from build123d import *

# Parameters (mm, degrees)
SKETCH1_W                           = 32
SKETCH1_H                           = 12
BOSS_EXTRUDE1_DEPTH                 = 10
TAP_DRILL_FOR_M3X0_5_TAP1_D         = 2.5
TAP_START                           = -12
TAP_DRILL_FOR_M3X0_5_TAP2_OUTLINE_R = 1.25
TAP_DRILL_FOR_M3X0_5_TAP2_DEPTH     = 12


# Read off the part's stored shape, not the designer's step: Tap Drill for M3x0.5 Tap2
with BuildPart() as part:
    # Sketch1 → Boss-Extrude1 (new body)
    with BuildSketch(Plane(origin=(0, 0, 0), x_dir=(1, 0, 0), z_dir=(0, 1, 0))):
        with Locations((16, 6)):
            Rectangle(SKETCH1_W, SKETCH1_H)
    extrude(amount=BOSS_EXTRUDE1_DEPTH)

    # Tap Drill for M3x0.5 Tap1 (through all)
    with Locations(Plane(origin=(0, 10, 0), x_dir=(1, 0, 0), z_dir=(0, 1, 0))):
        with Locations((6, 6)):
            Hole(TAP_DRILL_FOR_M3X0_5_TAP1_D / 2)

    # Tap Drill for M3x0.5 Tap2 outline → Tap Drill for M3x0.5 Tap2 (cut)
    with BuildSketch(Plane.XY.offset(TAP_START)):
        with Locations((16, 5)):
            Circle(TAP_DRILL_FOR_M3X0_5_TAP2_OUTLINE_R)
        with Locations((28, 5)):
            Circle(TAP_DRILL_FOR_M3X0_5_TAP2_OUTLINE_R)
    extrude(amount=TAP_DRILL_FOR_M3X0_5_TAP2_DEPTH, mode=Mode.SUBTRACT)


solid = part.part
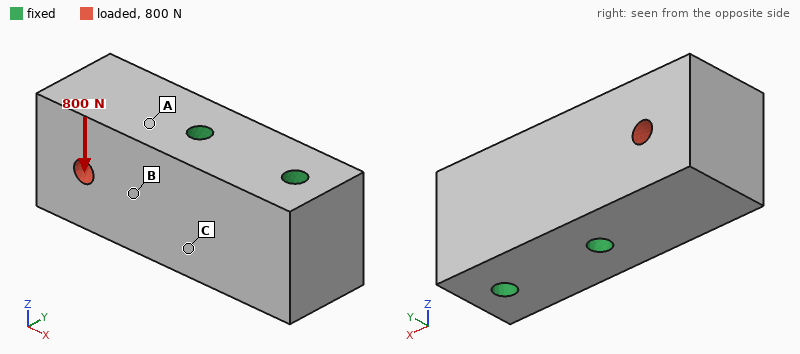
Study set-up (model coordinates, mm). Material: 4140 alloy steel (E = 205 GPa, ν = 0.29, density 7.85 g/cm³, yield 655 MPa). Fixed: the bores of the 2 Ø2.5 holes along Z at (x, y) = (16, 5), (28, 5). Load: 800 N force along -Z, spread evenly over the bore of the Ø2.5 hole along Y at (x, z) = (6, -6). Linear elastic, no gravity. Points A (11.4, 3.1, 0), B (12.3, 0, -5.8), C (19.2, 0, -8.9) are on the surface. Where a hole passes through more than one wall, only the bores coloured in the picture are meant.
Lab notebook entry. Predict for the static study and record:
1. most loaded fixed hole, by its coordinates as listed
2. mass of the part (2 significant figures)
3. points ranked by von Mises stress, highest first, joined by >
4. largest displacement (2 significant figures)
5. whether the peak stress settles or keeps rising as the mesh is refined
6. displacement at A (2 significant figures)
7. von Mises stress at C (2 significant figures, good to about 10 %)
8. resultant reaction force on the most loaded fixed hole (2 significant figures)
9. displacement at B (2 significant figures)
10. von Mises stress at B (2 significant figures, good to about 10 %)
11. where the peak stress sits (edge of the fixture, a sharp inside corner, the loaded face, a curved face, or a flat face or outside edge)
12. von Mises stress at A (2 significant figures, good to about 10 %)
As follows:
(16, 5)
29 g
A > B > C
3.2 µm
keeps rising
1.1 µm
5.1 MPa
870 N
0.55 µm
13 MPa
edge of the fixture
20 MPa
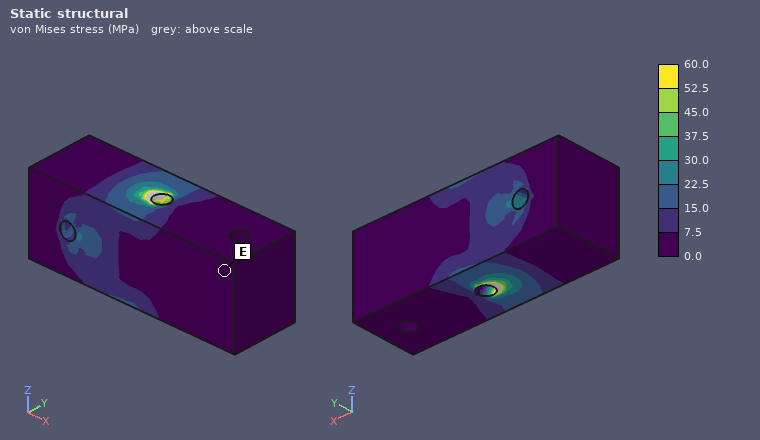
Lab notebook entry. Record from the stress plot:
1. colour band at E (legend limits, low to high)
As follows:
0.0 to 7.5 MPa
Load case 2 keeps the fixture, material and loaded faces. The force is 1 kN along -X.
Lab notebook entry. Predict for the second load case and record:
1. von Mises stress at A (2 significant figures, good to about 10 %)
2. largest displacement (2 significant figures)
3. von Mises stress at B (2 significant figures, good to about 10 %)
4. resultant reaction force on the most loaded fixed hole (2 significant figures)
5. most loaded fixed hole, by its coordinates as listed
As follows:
7.6 MPa
0.68 µm
7.3 MPa
880 N
(16, 5)
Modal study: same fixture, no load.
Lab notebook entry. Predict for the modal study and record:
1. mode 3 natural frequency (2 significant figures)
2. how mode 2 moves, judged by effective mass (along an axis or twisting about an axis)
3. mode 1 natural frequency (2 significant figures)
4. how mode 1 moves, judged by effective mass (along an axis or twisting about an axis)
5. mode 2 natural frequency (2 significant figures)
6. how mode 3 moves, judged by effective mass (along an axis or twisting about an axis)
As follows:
44 kHz
along Z
20 kHz
along Y
27 kHz
twisting about X
